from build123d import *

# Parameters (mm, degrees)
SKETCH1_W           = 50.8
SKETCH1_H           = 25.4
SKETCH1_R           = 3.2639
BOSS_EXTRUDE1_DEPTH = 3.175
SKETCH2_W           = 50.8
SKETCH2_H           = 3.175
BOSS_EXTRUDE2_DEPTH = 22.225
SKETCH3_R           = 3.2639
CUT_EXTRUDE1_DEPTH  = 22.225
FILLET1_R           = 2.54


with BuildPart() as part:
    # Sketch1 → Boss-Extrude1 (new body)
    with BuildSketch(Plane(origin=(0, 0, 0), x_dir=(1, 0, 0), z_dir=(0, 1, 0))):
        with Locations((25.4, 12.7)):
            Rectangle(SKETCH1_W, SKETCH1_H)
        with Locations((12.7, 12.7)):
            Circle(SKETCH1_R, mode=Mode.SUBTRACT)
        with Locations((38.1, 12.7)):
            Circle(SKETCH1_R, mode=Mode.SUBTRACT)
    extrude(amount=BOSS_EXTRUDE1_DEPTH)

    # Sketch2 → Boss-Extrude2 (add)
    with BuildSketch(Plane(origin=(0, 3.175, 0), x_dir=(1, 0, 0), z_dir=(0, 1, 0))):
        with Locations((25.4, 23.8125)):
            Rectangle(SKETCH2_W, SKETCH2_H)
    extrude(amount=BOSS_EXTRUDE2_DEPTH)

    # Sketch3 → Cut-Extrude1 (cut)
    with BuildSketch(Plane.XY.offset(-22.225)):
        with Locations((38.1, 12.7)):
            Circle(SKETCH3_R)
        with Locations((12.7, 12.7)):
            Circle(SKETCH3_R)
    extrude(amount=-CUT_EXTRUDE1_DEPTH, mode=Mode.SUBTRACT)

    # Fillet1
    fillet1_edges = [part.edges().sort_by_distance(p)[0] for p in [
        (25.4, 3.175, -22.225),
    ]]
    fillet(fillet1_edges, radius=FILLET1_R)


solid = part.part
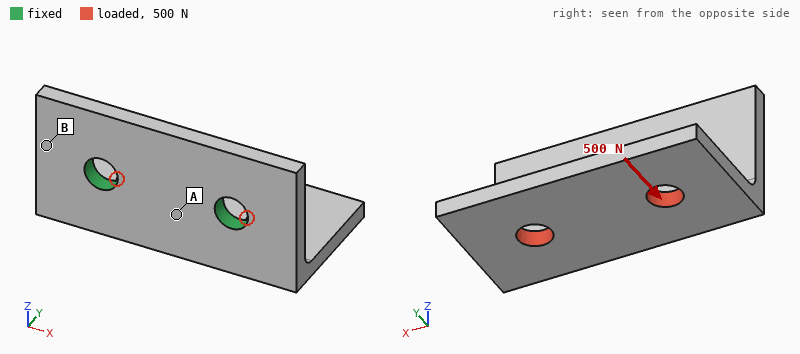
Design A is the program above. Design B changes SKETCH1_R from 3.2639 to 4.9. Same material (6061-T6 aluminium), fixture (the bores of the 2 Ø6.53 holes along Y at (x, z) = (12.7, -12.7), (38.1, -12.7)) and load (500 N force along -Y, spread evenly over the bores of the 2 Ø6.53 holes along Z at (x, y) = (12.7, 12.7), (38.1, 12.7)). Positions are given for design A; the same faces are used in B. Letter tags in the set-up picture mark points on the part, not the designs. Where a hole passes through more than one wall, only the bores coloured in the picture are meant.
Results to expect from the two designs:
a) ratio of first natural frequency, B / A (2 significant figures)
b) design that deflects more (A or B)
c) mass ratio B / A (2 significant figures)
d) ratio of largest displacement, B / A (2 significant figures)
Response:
1.1
A
0.96
0.62
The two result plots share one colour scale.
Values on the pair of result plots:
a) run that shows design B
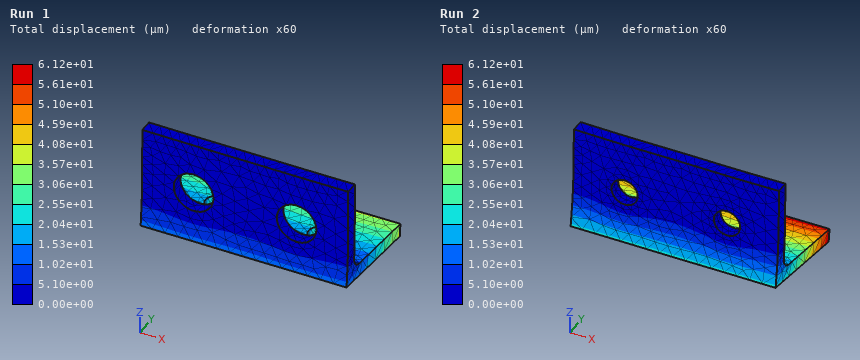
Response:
Run 1
